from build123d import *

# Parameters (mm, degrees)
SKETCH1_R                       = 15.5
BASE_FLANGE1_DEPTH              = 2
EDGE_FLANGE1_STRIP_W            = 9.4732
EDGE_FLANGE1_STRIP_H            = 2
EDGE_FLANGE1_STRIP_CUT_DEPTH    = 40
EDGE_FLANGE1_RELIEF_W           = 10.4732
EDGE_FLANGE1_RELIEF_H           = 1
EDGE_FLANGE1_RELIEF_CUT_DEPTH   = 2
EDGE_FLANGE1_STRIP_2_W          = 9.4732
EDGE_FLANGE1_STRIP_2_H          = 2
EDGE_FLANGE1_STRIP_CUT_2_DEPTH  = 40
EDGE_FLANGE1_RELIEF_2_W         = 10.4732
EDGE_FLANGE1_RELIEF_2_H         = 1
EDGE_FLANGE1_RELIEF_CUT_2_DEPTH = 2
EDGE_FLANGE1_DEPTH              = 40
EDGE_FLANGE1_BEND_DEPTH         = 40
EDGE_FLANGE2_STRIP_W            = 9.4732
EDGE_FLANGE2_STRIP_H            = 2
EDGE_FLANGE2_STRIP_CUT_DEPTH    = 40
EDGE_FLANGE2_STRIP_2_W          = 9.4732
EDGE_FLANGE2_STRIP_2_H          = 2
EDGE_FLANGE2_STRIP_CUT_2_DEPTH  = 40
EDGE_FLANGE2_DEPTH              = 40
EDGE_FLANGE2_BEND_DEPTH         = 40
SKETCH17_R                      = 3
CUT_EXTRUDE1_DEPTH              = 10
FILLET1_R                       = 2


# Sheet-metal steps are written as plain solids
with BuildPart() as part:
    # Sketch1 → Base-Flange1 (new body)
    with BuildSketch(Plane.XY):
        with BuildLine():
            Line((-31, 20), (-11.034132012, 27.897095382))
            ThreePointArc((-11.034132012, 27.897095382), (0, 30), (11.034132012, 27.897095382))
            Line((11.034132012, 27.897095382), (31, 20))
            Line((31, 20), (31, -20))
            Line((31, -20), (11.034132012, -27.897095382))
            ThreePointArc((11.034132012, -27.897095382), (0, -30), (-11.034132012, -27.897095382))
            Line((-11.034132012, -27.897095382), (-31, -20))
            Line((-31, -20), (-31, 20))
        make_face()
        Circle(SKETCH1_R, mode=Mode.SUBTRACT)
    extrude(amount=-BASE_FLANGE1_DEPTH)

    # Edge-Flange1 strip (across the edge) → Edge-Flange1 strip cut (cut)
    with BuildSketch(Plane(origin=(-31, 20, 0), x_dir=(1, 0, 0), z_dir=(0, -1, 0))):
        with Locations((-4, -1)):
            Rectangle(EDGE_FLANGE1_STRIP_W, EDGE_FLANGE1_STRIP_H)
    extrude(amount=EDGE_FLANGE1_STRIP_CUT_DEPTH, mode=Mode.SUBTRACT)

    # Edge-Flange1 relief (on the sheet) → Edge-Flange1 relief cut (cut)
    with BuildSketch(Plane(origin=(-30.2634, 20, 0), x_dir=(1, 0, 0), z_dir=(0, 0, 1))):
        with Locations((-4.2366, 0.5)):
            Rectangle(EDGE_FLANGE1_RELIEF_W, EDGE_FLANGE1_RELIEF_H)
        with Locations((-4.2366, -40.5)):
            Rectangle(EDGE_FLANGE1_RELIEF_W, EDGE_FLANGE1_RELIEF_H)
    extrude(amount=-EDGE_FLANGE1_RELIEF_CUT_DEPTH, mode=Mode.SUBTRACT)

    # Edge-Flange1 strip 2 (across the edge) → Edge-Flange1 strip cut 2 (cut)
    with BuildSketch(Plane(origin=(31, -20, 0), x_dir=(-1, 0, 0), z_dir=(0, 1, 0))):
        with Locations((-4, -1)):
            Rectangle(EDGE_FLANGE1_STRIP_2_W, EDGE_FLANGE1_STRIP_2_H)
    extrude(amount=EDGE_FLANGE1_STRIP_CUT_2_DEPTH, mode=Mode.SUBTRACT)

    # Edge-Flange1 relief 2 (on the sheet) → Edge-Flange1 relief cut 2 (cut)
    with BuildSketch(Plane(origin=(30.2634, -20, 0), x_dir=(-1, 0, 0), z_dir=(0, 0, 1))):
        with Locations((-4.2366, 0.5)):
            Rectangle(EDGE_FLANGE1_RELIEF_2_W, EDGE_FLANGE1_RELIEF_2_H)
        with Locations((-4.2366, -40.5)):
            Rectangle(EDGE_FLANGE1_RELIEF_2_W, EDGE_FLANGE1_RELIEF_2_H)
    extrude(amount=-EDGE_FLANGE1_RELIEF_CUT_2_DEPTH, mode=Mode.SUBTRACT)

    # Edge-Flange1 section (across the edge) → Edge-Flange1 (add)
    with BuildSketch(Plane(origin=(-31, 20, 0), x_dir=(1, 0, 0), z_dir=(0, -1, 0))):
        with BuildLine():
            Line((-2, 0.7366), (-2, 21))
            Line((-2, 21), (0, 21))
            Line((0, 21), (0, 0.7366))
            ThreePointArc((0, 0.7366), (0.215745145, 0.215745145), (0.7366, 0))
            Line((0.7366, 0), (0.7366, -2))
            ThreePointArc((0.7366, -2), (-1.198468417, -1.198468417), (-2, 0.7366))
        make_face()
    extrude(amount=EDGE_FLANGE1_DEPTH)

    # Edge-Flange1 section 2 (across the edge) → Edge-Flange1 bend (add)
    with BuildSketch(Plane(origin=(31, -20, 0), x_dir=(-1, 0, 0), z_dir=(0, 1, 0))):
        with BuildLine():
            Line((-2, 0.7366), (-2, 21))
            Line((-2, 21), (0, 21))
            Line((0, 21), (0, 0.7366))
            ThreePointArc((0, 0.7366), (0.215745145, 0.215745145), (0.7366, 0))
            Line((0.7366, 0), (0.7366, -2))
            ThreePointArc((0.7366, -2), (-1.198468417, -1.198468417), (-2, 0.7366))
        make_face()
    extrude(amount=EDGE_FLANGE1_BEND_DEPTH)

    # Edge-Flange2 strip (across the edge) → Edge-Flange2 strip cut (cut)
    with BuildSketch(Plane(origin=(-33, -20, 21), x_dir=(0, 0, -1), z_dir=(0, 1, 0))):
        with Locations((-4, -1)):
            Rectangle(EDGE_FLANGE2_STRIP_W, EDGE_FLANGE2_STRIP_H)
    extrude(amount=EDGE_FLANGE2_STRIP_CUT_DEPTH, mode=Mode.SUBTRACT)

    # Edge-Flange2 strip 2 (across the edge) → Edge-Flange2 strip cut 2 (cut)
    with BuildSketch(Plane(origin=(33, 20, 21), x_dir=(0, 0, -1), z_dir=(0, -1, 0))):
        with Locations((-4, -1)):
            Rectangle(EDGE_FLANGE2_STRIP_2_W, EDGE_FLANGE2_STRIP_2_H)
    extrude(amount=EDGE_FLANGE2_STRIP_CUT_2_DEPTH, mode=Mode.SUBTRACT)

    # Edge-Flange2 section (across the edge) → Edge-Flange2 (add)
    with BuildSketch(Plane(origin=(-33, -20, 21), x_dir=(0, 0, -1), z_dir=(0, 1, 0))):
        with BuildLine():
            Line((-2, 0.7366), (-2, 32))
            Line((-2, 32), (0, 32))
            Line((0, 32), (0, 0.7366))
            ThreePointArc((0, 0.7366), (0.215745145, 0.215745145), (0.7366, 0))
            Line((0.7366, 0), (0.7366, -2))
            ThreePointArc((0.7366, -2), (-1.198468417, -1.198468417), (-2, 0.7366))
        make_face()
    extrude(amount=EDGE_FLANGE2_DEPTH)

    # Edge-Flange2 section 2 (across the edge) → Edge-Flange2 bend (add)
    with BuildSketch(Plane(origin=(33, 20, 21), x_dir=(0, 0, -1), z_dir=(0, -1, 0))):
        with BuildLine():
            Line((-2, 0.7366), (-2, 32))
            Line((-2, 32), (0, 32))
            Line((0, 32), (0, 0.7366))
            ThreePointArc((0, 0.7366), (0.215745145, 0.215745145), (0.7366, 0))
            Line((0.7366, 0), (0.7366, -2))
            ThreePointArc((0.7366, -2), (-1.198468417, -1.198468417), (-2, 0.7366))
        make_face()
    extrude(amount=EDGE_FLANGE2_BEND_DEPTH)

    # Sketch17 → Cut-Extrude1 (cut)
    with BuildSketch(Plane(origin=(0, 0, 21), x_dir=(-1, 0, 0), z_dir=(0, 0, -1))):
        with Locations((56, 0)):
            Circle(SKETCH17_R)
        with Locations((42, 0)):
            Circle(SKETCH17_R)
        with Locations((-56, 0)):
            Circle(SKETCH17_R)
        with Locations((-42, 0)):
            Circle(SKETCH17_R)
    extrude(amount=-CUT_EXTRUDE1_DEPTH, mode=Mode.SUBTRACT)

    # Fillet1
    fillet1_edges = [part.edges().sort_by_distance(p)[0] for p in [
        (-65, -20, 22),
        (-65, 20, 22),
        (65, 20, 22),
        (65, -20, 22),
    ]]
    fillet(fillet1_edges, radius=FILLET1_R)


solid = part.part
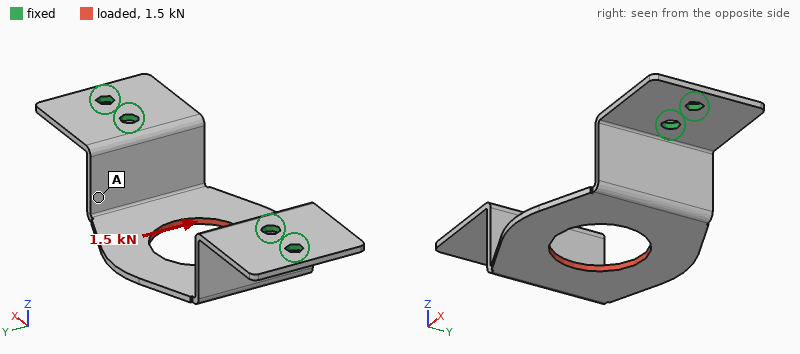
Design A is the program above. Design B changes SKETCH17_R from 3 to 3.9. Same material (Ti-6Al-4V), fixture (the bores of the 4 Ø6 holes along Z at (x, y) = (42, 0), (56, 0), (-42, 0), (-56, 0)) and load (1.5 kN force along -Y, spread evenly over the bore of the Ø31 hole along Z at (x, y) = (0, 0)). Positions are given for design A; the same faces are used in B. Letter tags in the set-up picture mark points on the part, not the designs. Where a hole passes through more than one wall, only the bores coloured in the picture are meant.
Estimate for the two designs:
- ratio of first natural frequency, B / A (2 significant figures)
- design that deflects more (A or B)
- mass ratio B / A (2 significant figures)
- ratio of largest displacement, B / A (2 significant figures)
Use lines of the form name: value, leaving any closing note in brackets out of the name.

ratio of first natural frequency, B / A: 1.1
design that deflects more: A
mass ratio B / A: 0.99
ratio of largest displacement, B / A: 0.78
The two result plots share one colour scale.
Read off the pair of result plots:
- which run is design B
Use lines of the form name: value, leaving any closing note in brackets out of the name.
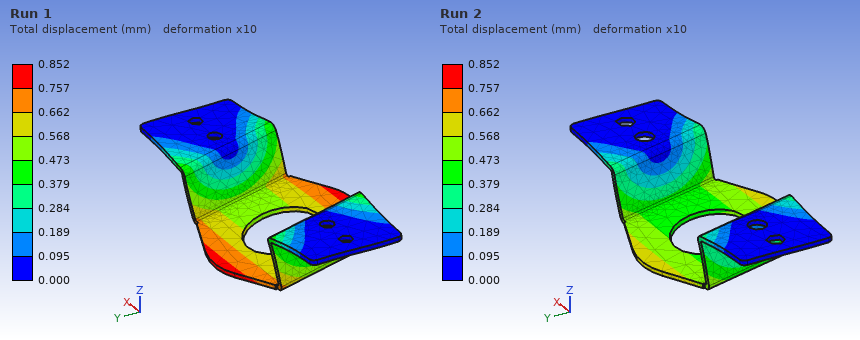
which run is design B: Run 2
